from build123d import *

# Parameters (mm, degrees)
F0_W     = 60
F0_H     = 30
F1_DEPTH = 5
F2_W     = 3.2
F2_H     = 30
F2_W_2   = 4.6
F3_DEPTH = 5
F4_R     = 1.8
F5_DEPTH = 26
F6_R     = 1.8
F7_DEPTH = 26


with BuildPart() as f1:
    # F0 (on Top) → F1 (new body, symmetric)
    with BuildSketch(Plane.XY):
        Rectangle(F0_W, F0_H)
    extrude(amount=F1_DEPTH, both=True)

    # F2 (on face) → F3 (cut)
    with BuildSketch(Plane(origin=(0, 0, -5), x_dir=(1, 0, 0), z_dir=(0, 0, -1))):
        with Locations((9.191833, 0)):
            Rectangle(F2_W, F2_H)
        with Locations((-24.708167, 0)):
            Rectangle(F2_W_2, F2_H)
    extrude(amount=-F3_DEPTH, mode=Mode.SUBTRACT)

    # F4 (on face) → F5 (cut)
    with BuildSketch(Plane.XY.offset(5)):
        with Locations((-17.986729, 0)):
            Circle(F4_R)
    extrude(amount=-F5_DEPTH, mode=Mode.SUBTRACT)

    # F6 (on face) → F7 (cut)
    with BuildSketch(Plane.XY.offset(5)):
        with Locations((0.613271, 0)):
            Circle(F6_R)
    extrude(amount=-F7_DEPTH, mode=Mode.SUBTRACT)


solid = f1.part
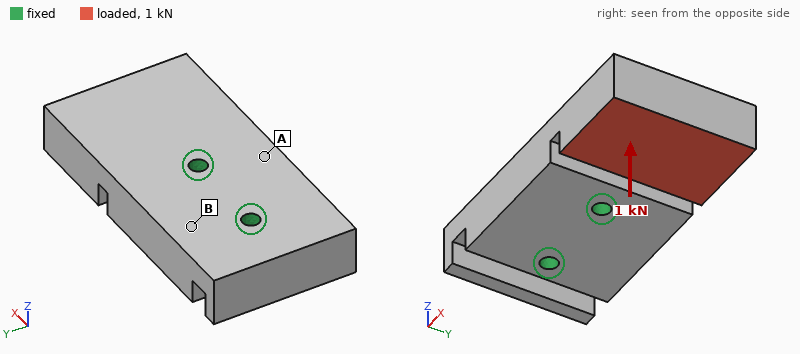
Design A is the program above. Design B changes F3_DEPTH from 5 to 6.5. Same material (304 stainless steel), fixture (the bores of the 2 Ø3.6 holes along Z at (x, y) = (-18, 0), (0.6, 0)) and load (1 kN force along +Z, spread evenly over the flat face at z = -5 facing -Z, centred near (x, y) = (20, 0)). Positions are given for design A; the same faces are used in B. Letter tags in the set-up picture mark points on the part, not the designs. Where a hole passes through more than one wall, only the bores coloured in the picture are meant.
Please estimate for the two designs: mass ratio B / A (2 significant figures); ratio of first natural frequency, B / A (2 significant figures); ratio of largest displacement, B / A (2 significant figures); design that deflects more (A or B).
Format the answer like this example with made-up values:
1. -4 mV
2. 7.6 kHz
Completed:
1. 0.98
2. 0.68
3. 2.2
4. B
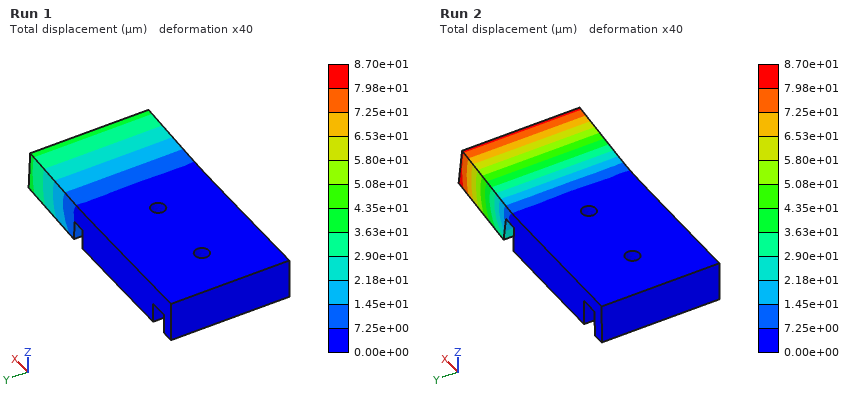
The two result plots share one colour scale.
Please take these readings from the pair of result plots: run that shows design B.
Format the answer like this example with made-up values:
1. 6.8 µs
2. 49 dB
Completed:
1. Run 2
